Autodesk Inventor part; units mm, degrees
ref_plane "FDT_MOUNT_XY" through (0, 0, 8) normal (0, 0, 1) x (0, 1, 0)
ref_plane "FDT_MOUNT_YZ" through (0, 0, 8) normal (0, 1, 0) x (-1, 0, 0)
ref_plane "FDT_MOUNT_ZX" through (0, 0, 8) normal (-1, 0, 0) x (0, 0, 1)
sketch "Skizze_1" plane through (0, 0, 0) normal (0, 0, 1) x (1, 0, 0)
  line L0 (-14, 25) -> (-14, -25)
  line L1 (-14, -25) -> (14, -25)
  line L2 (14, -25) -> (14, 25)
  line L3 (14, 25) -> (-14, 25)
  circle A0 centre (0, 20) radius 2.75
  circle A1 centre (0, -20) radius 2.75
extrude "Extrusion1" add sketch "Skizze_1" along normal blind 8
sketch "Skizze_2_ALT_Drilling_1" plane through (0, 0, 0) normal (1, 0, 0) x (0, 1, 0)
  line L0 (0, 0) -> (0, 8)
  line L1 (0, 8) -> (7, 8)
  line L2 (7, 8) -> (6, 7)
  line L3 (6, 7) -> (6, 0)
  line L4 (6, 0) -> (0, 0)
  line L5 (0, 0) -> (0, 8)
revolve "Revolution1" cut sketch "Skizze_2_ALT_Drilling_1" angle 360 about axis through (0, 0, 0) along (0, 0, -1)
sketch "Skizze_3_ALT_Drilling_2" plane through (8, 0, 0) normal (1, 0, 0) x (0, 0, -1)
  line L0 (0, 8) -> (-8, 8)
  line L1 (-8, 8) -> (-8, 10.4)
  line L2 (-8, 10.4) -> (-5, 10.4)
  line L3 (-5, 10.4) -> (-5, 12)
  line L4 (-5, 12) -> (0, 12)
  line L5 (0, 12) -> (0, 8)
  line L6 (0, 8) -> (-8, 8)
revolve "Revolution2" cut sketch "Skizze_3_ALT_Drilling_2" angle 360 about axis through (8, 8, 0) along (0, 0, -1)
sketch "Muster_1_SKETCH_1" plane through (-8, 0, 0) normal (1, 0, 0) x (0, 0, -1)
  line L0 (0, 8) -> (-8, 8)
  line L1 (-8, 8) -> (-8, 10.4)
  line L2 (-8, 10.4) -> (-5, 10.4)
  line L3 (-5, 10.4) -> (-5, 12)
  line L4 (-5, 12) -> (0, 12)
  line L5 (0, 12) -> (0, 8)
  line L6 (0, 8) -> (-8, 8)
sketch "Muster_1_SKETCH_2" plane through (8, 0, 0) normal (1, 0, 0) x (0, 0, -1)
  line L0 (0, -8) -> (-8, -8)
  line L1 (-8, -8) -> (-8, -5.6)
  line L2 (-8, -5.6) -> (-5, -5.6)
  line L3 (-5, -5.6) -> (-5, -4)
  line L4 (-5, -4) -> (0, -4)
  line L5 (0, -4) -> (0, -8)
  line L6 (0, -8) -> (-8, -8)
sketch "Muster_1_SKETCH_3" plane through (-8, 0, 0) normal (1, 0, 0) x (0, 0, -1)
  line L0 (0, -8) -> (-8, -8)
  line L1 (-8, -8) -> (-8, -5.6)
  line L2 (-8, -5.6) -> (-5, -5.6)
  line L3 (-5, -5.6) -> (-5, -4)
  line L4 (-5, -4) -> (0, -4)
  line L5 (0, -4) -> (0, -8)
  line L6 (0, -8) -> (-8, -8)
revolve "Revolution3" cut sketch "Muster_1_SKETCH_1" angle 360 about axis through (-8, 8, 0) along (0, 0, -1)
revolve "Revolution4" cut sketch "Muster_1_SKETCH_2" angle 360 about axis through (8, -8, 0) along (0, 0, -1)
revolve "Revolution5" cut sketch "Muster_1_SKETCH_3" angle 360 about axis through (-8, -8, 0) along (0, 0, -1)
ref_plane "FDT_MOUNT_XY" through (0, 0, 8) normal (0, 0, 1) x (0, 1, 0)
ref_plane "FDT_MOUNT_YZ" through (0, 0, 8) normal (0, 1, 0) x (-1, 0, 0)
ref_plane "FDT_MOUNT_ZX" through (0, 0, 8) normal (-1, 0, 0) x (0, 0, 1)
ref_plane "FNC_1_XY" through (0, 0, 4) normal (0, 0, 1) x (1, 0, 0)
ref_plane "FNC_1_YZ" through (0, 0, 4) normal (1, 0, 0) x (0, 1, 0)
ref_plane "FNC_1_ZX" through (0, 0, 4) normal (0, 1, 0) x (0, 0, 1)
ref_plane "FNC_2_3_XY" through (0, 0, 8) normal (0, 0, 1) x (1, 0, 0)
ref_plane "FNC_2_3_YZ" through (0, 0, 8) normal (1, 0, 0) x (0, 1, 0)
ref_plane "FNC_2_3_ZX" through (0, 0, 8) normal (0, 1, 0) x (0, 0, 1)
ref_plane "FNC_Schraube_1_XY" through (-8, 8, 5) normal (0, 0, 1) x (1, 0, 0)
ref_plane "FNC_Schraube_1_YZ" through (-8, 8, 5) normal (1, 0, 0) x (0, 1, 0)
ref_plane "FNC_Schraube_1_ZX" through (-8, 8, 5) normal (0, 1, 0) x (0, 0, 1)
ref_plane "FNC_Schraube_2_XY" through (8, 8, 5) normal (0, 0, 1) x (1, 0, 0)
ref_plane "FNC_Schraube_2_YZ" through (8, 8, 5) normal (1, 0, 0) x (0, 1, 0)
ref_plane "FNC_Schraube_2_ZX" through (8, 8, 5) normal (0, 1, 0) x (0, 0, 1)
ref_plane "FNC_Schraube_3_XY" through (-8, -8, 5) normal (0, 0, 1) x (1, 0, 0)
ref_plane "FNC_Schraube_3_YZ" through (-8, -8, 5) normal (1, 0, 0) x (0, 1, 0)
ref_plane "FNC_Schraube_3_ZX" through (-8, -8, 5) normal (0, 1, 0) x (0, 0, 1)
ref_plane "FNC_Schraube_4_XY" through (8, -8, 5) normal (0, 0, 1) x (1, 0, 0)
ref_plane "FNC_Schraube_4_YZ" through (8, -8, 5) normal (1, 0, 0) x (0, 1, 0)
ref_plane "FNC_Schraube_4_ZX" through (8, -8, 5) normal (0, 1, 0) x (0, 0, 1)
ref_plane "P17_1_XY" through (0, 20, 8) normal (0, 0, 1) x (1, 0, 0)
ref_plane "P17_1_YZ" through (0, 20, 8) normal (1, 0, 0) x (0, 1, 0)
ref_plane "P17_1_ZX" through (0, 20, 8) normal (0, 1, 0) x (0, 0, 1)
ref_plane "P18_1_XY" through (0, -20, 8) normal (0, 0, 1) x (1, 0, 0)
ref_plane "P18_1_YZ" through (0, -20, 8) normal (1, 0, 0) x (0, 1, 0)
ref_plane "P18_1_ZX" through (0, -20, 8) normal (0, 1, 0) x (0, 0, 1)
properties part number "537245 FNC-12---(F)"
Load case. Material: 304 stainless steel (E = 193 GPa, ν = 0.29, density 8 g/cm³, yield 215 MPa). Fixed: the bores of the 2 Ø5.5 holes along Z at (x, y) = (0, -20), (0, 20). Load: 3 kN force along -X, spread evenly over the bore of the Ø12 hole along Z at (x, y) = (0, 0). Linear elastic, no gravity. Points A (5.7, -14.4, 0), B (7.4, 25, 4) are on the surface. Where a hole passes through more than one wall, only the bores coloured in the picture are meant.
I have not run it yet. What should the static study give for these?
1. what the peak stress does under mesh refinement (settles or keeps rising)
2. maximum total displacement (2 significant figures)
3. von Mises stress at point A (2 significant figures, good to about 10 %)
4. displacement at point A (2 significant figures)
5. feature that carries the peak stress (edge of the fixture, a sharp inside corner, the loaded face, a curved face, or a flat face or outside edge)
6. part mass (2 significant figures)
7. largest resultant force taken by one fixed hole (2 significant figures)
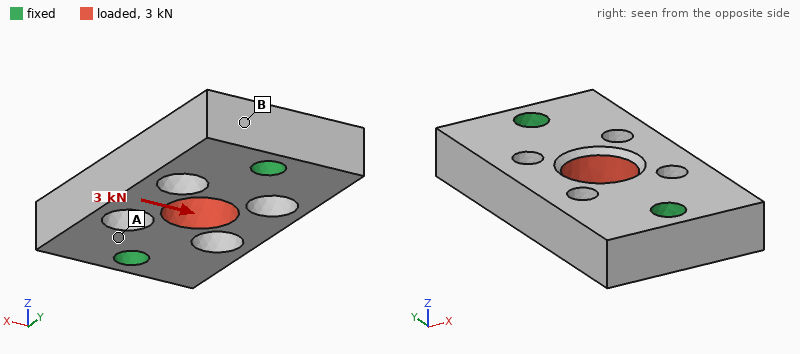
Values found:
keeps rising
5.2 µm
22 MPa
1.3 µm
a sharp inside corner
69 g
1.5 kN
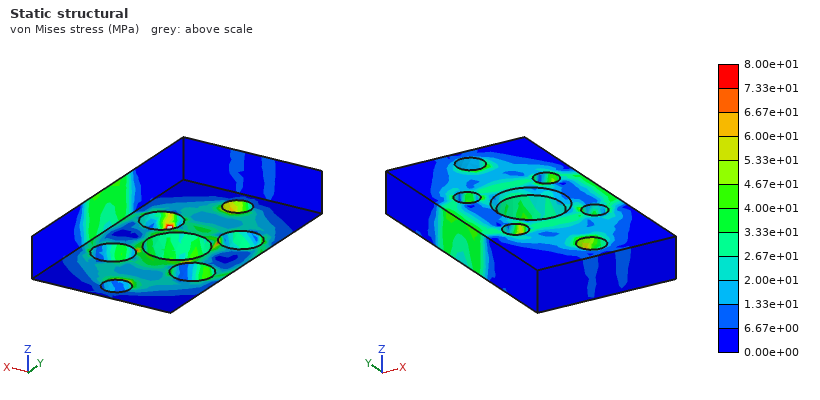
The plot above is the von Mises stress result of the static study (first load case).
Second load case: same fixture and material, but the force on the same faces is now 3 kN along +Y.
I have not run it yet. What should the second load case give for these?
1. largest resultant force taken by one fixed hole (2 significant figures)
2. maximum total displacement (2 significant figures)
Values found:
1.5 kN
2.7 µm
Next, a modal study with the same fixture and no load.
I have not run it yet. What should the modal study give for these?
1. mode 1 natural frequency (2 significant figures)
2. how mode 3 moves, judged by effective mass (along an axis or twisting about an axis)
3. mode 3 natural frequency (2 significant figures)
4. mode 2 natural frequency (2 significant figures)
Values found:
18 kHz
along X
28 kHz
18 kHz
